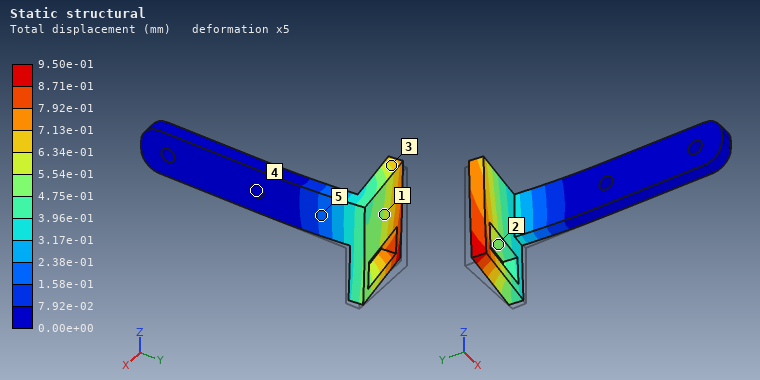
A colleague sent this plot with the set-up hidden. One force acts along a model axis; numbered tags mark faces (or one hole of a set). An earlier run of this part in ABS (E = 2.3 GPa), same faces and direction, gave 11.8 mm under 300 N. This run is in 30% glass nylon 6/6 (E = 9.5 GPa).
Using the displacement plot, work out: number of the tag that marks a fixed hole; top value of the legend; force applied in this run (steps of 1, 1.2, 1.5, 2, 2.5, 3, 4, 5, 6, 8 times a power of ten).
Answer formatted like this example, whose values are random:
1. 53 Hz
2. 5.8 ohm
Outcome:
1. 4
2. 9.50e-01 mm
3. 100 N
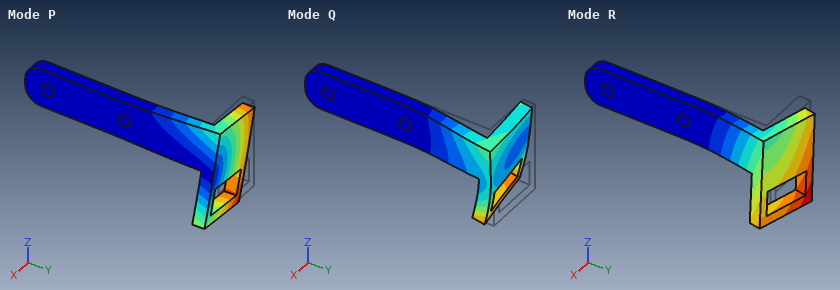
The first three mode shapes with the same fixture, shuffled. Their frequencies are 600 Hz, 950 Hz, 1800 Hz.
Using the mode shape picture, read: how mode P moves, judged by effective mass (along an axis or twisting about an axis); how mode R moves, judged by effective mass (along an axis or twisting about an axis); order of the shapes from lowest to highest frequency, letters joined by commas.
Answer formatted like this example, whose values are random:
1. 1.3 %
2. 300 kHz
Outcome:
1. along Z
2. along X
3. R, P, Q
